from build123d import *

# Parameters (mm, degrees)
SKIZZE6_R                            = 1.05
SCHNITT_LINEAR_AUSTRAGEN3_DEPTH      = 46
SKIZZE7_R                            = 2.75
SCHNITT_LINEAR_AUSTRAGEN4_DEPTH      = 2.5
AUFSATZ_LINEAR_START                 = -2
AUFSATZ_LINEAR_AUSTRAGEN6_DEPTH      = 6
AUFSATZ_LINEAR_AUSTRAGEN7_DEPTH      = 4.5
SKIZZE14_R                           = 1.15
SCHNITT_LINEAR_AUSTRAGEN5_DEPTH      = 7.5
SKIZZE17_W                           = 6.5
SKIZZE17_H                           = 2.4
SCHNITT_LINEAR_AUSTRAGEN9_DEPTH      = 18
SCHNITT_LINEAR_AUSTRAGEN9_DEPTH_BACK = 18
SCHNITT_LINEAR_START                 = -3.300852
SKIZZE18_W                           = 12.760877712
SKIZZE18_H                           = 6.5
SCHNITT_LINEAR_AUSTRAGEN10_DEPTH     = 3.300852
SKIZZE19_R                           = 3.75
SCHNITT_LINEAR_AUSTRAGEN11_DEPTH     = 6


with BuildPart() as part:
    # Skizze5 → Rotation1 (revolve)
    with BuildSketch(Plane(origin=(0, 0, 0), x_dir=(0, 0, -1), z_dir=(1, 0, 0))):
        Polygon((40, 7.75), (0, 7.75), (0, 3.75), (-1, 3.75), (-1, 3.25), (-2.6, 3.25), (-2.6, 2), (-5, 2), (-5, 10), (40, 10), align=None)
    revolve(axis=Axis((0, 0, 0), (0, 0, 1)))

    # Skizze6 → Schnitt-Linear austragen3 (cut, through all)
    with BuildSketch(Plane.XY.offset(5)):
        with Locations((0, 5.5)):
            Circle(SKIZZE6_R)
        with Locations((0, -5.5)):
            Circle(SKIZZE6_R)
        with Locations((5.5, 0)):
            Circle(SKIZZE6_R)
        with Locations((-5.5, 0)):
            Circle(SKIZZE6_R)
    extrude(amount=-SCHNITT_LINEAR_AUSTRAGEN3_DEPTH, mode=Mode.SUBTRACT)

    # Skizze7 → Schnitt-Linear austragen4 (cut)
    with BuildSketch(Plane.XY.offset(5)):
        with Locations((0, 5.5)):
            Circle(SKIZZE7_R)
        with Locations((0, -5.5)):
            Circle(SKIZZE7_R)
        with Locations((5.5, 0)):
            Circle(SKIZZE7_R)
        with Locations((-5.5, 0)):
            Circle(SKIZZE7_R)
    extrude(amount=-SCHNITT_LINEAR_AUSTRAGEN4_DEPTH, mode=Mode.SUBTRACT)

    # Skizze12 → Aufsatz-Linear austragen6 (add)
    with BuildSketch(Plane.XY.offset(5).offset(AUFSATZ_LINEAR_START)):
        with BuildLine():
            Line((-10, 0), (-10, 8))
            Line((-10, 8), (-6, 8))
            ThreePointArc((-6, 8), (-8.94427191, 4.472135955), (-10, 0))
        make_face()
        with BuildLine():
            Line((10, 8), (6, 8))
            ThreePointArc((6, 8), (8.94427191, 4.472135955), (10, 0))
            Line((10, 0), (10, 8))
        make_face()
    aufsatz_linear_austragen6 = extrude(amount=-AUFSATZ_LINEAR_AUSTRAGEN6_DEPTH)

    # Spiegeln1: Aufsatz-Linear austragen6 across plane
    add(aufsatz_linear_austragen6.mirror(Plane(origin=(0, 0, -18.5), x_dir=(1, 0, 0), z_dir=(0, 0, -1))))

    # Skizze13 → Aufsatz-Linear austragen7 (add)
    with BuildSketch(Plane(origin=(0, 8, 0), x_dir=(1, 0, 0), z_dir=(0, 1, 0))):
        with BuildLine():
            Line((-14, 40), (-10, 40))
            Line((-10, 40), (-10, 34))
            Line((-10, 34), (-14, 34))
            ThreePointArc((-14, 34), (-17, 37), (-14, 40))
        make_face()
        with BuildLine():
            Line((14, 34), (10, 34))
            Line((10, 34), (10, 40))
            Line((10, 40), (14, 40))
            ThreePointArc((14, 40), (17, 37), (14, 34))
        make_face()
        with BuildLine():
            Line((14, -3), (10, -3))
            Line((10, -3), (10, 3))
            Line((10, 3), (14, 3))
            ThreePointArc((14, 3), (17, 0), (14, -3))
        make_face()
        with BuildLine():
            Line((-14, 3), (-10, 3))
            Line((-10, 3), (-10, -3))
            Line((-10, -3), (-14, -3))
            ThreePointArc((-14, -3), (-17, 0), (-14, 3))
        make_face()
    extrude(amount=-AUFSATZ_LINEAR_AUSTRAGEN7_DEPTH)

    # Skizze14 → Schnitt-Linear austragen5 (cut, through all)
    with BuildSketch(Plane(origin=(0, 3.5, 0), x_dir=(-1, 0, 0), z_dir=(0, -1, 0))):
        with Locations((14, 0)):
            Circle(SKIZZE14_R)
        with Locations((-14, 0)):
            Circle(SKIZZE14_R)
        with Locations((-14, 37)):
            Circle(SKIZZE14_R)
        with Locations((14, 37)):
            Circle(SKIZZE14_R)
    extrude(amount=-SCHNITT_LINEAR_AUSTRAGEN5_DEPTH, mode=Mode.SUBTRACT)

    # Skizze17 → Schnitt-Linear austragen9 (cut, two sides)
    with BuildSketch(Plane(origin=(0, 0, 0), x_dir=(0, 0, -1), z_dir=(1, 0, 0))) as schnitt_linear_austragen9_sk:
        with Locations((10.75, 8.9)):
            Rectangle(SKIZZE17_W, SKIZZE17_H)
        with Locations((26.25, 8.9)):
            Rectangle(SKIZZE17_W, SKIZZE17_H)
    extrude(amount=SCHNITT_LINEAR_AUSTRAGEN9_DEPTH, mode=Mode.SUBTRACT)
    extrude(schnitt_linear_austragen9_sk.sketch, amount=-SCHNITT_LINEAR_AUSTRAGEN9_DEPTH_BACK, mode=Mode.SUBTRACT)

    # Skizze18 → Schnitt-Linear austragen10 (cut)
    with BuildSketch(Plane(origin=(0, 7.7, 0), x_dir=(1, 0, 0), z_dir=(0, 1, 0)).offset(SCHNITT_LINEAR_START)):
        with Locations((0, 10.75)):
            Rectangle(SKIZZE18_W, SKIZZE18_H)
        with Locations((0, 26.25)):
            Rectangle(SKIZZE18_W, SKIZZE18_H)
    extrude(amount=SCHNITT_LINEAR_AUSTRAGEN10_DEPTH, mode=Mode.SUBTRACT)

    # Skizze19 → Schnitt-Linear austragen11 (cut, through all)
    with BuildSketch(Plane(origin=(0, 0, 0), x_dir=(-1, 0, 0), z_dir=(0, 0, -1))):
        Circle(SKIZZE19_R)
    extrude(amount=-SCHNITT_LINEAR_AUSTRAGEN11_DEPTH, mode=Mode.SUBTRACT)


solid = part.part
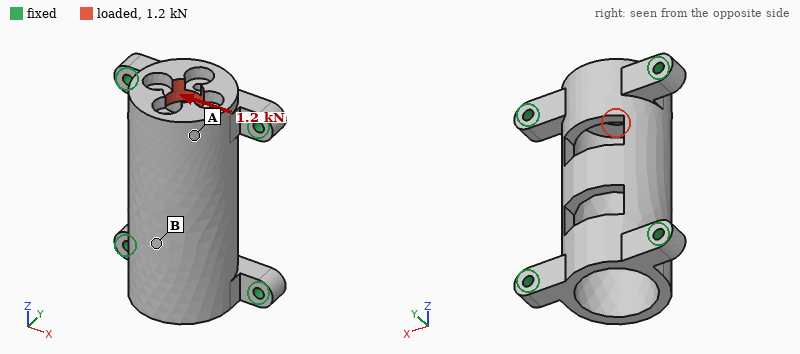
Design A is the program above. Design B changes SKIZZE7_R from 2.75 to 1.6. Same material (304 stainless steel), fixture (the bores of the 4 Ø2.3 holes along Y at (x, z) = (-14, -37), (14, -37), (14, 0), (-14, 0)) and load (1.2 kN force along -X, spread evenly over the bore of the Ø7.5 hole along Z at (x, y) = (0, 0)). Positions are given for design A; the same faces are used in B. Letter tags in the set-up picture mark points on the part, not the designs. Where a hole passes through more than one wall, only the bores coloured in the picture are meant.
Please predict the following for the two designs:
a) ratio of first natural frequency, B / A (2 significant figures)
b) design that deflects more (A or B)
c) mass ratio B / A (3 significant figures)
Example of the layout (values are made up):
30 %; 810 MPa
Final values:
1.0; A; 1.02
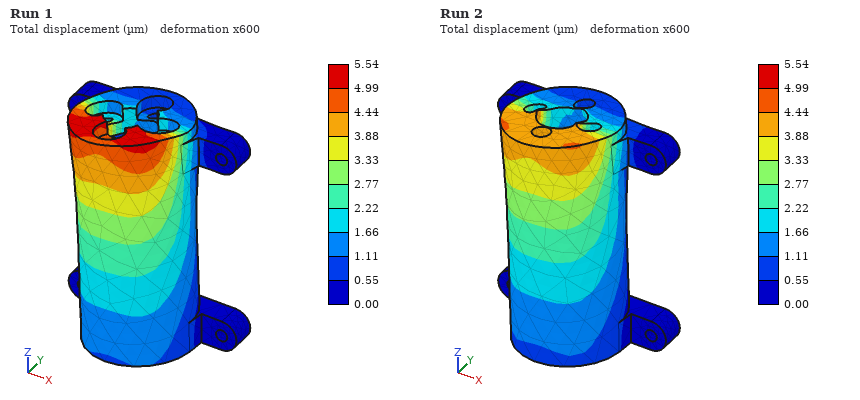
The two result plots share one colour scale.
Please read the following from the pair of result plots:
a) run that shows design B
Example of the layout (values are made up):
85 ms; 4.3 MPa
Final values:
Run 2
